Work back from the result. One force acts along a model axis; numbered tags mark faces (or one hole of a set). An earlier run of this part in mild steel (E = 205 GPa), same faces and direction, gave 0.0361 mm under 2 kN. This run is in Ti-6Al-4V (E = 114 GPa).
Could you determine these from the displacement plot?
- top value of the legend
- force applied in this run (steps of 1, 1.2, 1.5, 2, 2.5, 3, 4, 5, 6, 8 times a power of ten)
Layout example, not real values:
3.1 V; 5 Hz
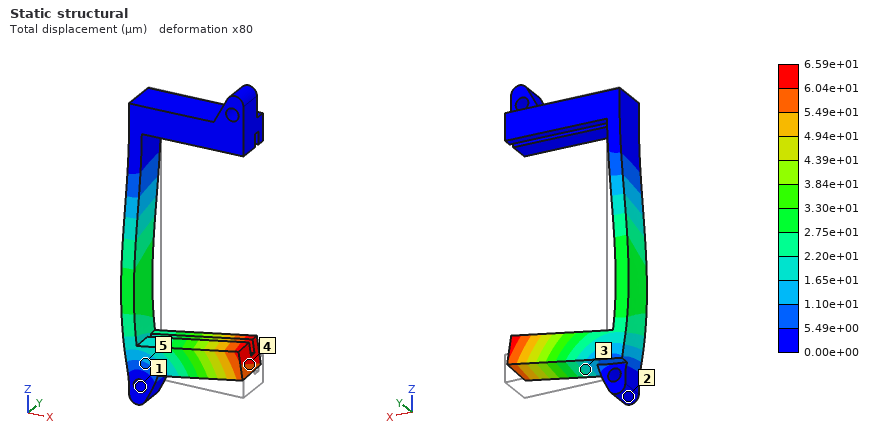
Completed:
6.59e+01 µm; 2 kN
